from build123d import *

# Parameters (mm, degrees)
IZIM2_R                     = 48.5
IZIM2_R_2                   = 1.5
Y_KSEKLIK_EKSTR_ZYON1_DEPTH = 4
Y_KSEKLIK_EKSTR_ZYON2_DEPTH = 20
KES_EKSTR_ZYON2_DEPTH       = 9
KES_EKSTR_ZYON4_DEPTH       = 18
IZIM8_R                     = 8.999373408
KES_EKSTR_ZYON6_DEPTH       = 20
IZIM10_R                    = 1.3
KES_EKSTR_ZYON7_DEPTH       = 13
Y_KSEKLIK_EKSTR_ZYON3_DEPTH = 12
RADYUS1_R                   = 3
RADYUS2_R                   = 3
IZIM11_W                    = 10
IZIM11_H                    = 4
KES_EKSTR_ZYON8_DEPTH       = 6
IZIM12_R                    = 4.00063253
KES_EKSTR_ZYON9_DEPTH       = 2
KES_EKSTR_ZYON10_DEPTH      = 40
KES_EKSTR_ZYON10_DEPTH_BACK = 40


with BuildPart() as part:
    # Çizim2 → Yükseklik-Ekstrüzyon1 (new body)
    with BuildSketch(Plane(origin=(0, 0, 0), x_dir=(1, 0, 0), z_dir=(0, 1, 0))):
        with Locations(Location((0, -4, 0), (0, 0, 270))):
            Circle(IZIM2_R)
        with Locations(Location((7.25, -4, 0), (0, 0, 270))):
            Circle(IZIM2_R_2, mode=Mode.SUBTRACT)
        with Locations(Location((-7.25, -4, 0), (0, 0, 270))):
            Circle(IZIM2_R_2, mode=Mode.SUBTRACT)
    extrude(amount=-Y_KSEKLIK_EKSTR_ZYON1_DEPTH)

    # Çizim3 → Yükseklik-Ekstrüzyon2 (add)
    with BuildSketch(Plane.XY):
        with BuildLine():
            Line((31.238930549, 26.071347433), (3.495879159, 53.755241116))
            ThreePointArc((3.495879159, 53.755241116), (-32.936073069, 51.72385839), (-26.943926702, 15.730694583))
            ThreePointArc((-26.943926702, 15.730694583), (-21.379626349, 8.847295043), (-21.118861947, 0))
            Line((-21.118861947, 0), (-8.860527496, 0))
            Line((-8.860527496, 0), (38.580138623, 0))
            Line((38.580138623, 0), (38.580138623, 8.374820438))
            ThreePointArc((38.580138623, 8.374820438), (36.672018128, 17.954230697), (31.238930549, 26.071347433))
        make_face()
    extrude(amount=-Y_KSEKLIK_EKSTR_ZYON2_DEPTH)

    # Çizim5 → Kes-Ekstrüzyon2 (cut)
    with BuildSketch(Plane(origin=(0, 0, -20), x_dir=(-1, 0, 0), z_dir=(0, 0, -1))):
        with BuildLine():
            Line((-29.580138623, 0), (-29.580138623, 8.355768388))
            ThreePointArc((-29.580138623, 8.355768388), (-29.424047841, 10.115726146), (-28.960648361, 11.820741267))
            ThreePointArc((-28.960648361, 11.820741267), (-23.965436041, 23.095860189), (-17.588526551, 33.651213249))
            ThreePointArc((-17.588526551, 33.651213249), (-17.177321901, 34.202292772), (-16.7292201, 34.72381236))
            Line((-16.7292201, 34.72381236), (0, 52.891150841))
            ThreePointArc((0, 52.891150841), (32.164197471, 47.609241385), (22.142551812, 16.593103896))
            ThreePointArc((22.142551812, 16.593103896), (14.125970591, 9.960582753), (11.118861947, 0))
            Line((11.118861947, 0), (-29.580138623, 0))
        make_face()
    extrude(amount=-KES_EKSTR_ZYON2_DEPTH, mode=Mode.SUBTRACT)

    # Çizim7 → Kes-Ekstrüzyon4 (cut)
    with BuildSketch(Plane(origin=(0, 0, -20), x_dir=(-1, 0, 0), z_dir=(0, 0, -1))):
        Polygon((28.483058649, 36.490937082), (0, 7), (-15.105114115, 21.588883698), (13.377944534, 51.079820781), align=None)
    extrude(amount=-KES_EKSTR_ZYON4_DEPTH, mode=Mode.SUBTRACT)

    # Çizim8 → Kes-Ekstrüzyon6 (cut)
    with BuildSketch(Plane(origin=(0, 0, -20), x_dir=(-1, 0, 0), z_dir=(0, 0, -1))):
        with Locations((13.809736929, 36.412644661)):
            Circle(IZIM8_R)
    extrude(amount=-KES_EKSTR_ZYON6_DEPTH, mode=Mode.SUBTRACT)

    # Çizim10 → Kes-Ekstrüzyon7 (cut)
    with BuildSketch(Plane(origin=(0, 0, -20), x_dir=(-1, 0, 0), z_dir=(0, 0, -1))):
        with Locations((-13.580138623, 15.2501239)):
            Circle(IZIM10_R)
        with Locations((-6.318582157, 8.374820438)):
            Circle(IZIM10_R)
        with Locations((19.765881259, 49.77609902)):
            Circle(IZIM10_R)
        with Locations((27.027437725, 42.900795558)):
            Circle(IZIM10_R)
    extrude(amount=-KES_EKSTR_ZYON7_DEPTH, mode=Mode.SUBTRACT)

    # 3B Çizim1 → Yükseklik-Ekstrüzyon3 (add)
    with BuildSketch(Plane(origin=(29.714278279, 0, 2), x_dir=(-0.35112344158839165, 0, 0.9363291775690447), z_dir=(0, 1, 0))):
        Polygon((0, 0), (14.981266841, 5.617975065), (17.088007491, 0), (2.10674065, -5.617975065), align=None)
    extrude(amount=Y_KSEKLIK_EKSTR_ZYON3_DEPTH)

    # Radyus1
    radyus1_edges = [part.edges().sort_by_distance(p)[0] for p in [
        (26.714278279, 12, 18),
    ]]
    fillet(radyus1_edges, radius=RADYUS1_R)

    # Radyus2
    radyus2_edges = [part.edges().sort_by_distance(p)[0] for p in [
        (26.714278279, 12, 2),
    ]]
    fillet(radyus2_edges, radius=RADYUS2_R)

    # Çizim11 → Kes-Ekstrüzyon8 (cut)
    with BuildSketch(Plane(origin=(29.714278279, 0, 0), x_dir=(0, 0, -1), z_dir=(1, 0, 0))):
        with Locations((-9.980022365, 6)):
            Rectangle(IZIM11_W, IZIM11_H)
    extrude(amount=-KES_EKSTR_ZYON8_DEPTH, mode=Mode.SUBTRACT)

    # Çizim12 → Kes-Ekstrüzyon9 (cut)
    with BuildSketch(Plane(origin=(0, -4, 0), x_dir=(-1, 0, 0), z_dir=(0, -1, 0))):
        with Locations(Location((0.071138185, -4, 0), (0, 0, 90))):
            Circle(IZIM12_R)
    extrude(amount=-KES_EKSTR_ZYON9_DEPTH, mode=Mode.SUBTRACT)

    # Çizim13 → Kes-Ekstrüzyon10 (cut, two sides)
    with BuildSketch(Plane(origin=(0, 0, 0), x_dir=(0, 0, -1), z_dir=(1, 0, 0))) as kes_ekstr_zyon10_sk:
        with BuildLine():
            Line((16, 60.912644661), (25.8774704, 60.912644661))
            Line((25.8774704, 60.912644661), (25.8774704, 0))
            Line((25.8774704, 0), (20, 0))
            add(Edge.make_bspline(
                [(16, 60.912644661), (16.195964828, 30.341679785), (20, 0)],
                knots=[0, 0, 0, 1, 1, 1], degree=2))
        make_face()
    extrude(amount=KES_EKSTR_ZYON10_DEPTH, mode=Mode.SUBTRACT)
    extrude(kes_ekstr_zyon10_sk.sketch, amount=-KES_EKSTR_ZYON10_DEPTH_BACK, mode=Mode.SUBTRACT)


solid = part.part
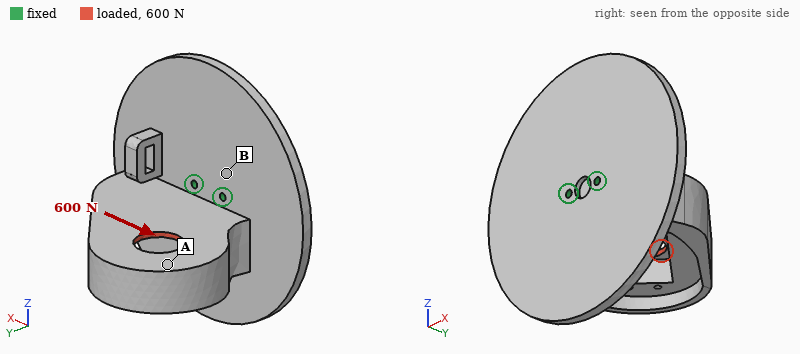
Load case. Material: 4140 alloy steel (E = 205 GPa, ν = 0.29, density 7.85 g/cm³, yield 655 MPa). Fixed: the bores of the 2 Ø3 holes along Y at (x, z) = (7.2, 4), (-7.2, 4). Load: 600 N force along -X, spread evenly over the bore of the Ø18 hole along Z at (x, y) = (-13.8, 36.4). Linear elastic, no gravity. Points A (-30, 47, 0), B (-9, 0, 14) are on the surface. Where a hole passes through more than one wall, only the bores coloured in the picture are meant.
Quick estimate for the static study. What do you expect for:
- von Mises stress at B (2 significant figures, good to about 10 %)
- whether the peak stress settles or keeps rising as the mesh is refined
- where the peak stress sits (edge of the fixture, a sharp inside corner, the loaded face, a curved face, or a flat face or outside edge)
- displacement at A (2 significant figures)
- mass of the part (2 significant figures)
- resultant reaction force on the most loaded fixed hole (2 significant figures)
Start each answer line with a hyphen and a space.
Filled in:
- 15 MPa
- keeps rising
- edge of the fixture
- 32 µm
- 500 g
- 1.3 kN
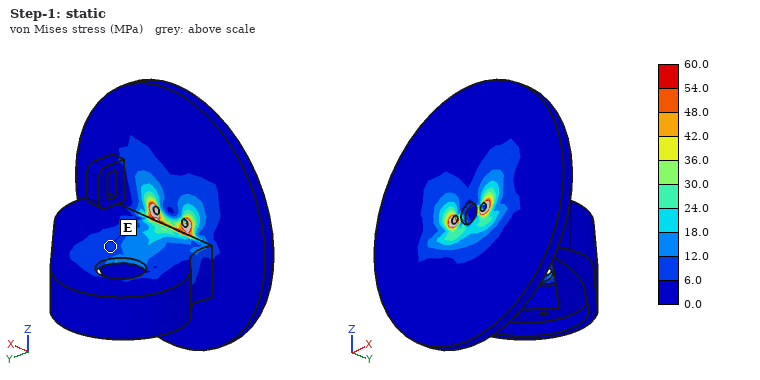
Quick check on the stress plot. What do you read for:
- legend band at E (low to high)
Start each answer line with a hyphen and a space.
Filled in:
- 6.0 to 12.0 MPa
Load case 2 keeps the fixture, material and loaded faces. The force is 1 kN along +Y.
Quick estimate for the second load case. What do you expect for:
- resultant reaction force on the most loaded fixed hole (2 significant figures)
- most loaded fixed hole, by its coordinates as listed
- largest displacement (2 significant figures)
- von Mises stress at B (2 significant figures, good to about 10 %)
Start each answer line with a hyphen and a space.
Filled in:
- 1.2 kN
- (-7.2, 4)
- 31 µm
- 11 MPa
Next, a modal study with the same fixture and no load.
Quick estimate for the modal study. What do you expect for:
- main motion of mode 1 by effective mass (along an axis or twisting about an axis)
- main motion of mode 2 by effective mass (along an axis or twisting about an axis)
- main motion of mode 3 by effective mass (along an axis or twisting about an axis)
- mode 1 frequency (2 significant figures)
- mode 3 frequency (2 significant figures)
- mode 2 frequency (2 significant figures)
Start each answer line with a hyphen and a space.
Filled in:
- along Z
- along X
- along Y
- 660 Hz
- 1700 Hz
- 1400 Hz
